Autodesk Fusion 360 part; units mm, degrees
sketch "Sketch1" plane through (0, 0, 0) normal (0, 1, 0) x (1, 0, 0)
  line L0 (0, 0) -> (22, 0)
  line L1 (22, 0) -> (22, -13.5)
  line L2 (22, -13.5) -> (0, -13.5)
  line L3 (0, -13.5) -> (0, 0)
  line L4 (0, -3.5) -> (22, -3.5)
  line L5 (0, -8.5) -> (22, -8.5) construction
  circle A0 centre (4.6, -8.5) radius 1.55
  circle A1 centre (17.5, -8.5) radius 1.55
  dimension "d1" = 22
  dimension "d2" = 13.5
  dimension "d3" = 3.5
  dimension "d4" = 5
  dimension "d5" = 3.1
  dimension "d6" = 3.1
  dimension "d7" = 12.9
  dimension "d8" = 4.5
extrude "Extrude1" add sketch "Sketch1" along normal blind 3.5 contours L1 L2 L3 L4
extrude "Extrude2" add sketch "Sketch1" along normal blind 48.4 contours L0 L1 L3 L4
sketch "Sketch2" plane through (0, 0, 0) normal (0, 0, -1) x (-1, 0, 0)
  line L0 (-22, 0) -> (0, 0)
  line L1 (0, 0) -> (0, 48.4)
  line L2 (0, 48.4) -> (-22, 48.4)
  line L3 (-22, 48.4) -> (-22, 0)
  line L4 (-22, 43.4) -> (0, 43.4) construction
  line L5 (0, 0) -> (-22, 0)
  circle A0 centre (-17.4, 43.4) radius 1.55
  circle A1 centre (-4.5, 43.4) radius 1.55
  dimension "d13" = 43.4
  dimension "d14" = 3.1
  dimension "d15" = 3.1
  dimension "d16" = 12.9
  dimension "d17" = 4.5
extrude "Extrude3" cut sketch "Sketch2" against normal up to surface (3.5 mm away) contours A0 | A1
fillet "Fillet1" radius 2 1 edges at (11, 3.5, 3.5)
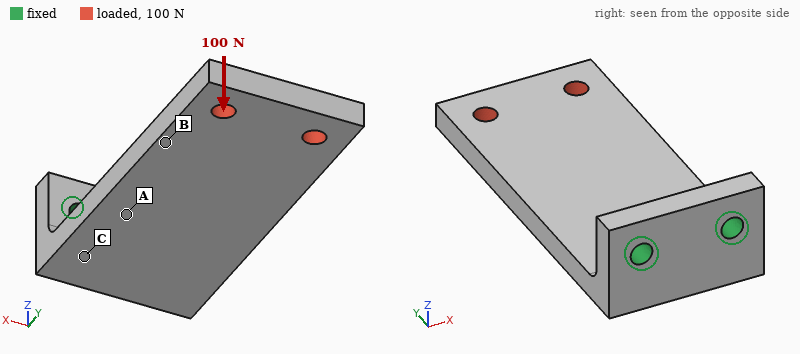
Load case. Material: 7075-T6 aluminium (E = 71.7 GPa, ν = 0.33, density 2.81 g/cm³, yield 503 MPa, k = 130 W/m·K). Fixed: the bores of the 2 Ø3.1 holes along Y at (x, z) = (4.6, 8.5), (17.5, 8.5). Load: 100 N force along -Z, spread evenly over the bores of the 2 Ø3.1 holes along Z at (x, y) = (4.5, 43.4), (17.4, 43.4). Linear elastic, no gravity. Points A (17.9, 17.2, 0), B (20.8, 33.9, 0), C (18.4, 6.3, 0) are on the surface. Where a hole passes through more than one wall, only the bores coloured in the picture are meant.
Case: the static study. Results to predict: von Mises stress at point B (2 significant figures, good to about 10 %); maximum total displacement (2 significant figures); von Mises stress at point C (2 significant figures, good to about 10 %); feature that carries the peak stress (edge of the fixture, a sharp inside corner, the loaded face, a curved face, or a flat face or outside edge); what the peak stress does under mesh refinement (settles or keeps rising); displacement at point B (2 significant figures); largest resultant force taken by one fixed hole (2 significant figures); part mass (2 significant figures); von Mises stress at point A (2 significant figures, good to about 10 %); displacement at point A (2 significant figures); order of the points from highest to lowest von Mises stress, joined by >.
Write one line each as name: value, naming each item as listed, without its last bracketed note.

von Mises stress at point B: 22 MPa
maximum total displacement: 0.61 mm
von Mises stress at point C: 78 MPa
feature that carries the peak stress: edge of the fixture
what the peak stress does under mesh refinement: keeps rising
displacement at point B: 0.36 mm
largest resultant force taken by one fixed hole: 76 N
part mass: 12 g
von Mises stress at point A: 57 MPa
displacement at point A: 0.12 mm
order of the points from highest to lowest von Mises stress, joined by >: C > A > B
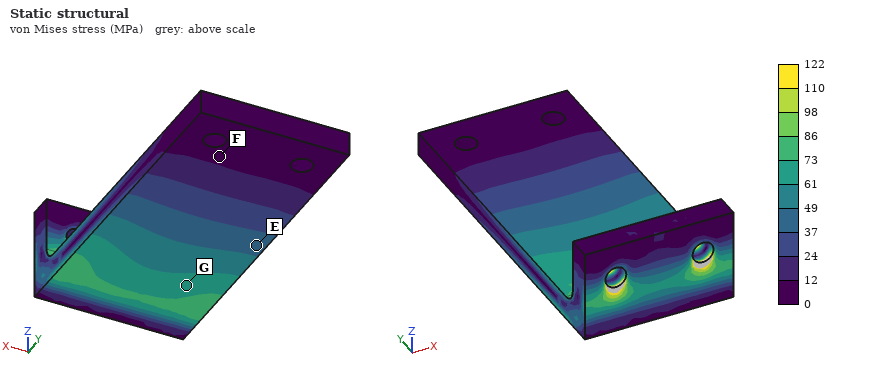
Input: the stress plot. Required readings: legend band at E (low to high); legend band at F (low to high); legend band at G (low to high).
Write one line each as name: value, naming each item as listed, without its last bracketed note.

legend band at E: 37 to 49 MPa
legend band at F: 0 to 12 MPa
legend band at G: 61 to 73 MPa
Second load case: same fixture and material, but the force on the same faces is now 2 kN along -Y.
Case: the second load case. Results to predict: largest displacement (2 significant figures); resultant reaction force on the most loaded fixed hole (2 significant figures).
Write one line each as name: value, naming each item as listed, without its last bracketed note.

largest displacement: 0.34 mm
resultant reaction force on the most loaded fixed hole: 1.0 kN
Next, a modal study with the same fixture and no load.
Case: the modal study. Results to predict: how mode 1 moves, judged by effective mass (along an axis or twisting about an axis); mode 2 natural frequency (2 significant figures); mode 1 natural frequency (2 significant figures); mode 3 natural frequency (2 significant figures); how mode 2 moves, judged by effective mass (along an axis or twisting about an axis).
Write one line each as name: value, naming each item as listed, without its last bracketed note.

how mode 1 moves, judged by effective mass: along Z
mode 2 natural frequency: 3700 Hz
mode 1 natural frequency: 1200 Hz
mode 3 natural frequency: 5800 Hz
how mode 2 moves, judged by effective mass: along X
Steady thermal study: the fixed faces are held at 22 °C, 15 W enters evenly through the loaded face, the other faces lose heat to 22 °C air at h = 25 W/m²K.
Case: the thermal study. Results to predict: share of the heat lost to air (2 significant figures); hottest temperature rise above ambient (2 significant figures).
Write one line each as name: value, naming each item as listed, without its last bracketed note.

share of the heat lost to air: 15 %
hottest temperature rise above ambient: 65 K
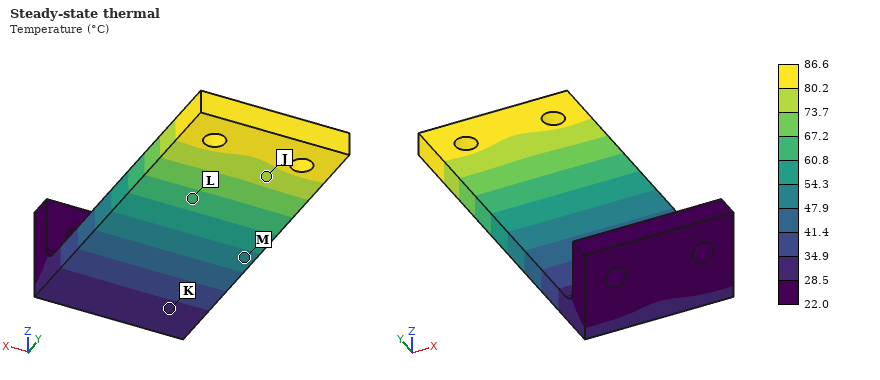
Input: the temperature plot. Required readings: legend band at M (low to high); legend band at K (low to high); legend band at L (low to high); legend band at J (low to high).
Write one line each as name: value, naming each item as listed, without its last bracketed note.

legend band at M: 47.9 to 54.3 °C
legend band at K: 28.5 to 34.9 °C
legend band at L: 60.8 to 67.2 °C
legend band at J: 73.7 to 80.2 °C
